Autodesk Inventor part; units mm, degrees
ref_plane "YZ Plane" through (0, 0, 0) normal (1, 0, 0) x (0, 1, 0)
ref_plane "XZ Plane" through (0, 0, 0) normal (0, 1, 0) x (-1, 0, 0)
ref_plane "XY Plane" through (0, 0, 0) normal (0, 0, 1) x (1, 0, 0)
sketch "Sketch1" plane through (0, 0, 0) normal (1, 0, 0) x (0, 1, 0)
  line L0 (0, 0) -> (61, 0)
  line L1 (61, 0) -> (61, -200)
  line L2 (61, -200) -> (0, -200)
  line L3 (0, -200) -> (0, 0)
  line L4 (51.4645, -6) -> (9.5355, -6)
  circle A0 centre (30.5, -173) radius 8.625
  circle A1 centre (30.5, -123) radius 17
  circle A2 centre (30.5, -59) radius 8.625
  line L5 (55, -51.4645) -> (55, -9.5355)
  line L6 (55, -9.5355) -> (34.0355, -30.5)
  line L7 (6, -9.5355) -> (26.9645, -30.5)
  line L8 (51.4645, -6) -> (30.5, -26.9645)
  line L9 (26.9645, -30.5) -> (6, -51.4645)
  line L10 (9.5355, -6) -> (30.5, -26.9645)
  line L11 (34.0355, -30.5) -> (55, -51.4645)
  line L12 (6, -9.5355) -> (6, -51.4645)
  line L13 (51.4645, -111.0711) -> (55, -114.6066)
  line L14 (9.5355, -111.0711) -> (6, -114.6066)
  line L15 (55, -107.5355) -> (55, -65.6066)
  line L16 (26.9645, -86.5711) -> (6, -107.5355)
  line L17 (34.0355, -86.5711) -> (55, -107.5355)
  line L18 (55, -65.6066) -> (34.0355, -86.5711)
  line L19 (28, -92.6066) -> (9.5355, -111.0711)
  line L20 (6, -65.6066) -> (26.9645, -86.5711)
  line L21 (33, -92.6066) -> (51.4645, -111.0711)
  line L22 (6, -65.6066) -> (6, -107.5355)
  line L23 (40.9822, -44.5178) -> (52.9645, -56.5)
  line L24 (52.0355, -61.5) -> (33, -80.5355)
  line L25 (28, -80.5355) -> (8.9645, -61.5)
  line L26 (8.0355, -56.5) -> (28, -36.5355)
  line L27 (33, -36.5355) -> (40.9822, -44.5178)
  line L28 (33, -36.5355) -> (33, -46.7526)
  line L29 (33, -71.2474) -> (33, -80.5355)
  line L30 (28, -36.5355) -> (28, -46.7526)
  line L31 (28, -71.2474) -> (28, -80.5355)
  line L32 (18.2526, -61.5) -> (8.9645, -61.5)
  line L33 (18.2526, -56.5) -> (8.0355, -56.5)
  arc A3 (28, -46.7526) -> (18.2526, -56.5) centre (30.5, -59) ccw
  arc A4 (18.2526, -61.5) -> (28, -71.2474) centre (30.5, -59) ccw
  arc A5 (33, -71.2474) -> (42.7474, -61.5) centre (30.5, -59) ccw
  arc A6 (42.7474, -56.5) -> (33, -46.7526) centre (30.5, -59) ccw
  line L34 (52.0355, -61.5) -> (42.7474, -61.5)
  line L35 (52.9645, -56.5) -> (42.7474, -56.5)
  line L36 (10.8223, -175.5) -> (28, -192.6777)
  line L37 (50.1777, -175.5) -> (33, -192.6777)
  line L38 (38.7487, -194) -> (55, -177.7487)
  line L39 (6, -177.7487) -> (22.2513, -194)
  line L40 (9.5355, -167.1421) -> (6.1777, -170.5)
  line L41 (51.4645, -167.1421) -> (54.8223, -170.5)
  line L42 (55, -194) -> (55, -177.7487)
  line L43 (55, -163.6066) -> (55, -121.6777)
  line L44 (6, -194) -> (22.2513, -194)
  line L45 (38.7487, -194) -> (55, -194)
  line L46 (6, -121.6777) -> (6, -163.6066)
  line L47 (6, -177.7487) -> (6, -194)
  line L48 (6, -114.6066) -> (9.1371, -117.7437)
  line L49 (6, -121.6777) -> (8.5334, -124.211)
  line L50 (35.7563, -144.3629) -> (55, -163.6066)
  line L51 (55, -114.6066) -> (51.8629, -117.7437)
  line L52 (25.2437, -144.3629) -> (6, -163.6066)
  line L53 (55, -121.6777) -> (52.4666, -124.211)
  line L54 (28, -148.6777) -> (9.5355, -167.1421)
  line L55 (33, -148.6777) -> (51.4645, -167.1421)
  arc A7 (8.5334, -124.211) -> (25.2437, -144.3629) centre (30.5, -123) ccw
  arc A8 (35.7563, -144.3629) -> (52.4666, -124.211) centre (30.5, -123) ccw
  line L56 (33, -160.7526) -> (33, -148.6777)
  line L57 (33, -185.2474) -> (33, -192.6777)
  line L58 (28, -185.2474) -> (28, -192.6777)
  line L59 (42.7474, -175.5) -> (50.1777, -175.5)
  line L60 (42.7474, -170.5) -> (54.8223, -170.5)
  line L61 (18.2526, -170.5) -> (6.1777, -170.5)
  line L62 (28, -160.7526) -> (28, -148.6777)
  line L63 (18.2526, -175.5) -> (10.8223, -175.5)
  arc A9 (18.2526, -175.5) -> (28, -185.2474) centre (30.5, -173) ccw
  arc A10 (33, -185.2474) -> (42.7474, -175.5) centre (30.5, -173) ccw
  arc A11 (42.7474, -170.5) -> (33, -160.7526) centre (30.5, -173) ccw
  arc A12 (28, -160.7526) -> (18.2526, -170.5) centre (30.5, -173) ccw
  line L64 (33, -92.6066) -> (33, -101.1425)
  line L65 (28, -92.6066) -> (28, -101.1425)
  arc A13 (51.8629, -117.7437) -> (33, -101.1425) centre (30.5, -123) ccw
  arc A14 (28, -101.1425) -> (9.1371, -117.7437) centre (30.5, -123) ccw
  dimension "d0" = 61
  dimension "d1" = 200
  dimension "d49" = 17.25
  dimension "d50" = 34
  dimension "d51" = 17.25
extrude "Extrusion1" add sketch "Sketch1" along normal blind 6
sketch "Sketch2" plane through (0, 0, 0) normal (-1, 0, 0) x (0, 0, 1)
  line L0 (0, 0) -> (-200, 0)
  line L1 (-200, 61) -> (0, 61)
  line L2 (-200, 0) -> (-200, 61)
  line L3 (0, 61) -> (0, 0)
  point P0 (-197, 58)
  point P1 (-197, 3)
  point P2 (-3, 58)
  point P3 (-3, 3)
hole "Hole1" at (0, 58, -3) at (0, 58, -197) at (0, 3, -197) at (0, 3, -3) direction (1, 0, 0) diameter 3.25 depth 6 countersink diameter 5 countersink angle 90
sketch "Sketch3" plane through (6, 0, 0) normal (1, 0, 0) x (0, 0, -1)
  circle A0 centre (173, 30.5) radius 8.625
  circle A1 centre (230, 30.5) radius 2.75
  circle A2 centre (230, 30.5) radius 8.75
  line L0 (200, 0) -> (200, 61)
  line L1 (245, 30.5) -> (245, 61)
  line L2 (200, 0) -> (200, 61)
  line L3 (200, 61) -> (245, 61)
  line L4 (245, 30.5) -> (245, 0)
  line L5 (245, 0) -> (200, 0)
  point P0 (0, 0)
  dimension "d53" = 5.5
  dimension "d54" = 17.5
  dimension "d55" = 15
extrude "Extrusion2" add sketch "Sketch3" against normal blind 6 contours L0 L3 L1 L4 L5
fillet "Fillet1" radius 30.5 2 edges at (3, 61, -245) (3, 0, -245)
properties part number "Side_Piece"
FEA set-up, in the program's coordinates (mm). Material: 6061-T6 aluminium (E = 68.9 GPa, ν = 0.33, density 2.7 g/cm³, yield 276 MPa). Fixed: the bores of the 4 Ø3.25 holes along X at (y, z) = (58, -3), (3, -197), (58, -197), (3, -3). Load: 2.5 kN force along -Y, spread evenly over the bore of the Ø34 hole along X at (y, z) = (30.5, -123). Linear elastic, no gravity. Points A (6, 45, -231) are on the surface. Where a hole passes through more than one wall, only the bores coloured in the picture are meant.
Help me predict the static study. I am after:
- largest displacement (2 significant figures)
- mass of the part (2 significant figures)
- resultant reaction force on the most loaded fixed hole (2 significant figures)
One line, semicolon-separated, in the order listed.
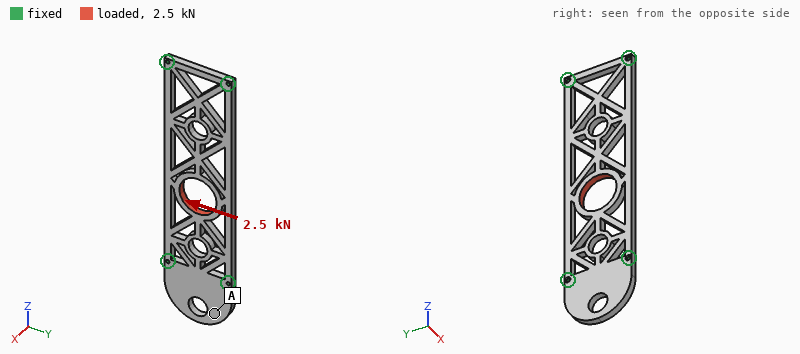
0.11 mm; 140 g; 1.3 kN
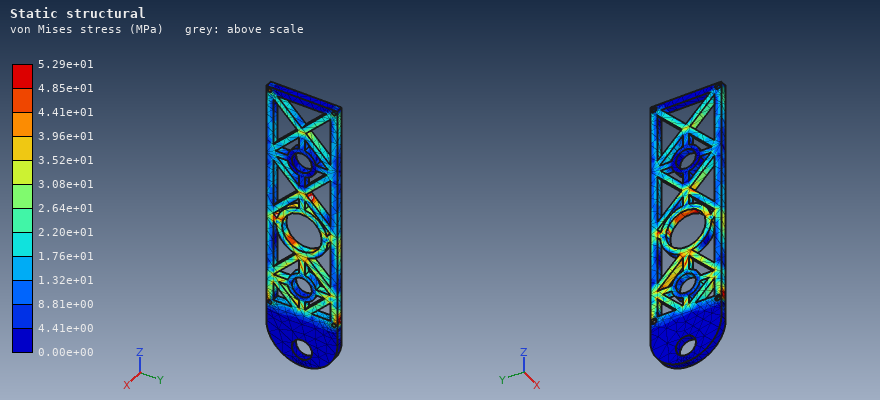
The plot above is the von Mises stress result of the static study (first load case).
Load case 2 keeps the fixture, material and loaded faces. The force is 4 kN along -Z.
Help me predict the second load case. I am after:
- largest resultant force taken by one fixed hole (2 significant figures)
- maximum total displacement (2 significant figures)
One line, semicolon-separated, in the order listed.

1.2 kN; 59 µm
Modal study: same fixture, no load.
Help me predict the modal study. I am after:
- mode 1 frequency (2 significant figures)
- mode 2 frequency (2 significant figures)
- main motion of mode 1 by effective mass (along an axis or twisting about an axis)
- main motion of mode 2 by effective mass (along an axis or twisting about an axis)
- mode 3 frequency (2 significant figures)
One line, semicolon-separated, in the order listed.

650 Hz; 1300 Hz; along X; twisting about Z; 1700 Hz
